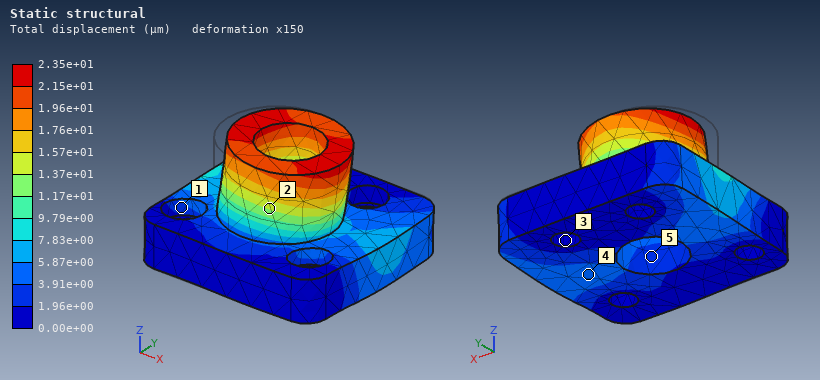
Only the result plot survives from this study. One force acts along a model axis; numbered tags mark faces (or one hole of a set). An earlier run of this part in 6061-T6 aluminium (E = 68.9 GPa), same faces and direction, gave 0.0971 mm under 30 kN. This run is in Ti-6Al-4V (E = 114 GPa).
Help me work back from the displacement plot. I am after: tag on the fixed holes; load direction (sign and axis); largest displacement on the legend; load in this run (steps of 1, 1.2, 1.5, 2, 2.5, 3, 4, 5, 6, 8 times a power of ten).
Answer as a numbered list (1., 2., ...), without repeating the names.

1. 3
2. +X
3. 2.35e+01 µm
4. 12 kN
